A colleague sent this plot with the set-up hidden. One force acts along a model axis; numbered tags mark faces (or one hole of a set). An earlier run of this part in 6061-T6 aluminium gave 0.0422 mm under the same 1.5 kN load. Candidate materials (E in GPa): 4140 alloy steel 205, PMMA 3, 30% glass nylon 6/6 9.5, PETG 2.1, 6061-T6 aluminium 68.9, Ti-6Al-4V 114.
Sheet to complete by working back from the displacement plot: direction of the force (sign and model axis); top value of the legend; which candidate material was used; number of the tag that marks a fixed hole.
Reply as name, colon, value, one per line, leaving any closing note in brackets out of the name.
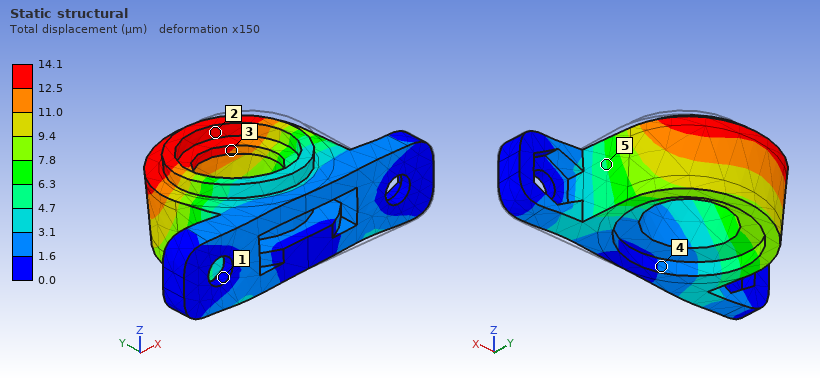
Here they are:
direction of the force: -X
top value of the legend: 14.1 µm
which candidate material was used: 4140 alloy steel
number of the tag that marks a fixed hole: 1
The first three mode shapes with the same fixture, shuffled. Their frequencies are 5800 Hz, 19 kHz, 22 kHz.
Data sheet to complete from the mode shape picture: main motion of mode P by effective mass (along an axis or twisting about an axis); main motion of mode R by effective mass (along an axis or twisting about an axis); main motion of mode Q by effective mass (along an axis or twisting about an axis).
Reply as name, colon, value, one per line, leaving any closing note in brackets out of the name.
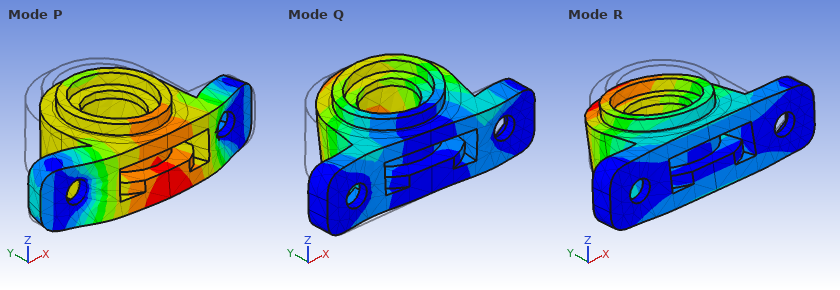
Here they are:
main motion of mode P by effective mass: along Y
main motion of mode R by effective mass: along Z
main motion of mode Q by effective mass: along X
